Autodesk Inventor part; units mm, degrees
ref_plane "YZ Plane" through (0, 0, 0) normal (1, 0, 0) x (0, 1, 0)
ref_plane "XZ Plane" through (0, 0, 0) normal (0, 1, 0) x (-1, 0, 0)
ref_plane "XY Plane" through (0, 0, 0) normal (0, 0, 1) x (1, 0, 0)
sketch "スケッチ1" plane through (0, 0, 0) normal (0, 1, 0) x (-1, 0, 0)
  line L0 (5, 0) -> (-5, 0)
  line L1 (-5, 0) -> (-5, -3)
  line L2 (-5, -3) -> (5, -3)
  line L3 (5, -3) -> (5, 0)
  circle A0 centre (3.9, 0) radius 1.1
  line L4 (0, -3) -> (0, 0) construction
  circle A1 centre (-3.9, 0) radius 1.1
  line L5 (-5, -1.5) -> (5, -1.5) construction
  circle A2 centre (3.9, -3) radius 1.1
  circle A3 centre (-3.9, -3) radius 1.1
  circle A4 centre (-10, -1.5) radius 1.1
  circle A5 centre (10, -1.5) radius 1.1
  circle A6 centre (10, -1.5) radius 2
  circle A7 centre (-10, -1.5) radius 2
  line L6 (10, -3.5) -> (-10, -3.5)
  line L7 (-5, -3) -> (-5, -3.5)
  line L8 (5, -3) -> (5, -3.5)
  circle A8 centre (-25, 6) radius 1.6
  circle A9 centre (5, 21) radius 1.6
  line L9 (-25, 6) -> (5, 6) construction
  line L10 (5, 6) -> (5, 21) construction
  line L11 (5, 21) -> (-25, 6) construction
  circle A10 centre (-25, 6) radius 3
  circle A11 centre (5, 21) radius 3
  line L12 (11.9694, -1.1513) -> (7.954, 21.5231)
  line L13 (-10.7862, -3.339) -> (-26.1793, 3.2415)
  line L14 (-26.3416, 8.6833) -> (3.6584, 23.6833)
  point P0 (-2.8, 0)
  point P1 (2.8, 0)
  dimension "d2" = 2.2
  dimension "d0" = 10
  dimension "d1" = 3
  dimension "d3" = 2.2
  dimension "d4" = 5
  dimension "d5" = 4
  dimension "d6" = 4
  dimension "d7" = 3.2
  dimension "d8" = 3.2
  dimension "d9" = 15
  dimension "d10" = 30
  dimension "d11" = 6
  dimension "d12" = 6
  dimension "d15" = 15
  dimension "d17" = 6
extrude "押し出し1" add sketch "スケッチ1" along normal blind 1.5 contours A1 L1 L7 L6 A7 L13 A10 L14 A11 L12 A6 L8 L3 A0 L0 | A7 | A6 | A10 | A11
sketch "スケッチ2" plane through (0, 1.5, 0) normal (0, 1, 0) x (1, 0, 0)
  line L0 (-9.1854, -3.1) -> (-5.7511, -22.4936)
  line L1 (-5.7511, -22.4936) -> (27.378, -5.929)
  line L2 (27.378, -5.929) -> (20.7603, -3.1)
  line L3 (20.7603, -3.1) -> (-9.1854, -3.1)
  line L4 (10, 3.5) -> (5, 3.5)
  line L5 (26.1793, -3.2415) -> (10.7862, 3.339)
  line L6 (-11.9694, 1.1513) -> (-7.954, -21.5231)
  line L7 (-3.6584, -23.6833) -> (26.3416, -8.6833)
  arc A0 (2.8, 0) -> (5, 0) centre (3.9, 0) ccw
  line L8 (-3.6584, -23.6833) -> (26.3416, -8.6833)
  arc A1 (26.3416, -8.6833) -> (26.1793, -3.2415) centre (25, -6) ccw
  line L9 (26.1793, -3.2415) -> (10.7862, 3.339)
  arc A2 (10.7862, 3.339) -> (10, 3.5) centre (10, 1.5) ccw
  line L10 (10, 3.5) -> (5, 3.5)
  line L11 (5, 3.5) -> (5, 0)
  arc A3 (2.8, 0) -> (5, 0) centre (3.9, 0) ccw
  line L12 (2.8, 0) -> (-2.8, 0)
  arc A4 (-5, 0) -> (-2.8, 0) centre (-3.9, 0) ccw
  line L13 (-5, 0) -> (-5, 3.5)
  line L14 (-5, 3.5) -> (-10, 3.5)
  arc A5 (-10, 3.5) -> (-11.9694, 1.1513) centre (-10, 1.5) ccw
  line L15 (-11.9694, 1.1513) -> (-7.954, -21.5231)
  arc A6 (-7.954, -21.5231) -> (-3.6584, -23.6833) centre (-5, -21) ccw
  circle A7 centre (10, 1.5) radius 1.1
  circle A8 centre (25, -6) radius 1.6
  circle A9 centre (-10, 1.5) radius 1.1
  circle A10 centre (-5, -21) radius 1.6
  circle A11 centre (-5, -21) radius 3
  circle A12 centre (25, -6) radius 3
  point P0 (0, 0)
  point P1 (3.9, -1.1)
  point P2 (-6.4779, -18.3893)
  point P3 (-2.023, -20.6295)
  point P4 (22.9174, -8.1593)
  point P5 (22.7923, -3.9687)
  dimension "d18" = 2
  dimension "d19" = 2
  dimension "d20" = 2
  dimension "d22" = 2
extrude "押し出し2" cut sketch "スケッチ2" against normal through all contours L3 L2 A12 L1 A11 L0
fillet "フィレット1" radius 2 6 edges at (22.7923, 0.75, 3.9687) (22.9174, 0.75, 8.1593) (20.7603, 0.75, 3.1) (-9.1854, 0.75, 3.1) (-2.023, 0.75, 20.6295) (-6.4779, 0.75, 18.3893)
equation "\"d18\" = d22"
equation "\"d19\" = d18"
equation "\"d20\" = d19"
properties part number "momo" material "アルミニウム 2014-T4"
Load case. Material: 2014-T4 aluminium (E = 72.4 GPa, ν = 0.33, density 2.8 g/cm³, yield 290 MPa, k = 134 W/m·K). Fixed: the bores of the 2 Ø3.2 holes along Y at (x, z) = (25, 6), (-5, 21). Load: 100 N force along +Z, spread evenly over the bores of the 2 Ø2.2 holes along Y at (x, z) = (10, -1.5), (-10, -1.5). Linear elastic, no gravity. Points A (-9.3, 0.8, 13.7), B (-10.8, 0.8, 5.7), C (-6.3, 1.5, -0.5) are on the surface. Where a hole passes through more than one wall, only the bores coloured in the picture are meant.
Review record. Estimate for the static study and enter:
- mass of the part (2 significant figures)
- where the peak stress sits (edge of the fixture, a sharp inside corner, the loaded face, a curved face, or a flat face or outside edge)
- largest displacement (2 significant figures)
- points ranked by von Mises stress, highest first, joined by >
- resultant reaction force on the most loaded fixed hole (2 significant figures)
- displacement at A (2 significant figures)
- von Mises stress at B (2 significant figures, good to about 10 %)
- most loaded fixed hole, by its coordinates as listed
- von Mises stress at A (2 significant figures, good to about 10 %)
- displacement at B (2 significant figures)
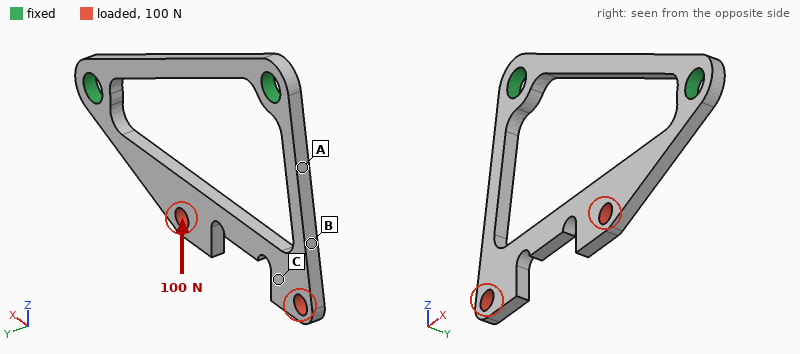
1.2 g
a curved face
73 µm
B > A > C
68 N
13 µm
64 MPa
(-5, 21)
25 MPa
22 µm
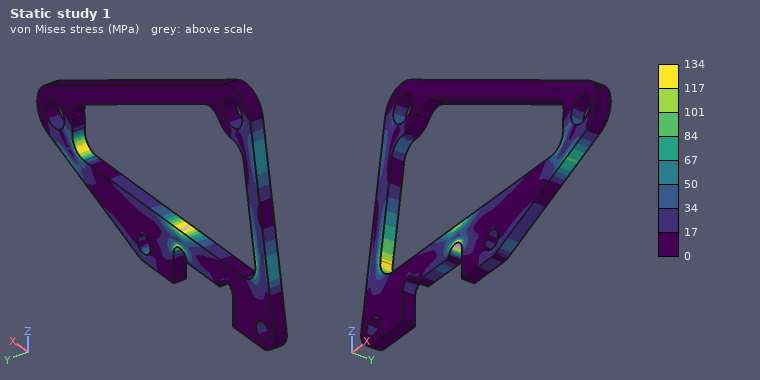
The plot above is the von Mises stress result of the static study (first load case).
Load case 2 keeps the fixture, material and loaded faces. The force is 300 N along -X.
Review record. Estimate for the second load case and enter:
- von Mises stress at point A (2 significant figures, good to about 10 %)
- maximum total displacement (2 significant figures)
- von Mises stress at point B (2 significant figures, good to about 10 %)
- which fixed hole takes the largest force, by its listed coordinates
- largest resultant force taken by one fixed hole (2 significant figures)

27 MPa
73 µm
61 MPa
(25, 6)
310 N
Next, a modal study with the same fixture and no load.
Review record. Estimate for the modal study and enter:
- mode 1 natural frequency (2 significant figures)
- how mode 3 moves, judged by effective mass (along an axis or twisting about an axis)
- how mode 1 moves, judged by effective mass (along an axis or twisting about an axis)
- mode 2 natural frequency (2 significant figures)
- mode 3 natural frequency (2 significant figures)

1700 Hz
along Z
along Y
4700 Hz
7500 Hz
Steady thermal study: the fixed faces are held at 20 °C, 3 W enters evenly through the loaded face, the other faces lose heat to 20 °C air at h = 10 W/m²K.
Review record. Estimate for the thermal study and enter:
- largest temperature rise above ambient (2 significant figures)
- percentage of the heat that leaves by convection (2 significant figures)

53 K
6.4 %
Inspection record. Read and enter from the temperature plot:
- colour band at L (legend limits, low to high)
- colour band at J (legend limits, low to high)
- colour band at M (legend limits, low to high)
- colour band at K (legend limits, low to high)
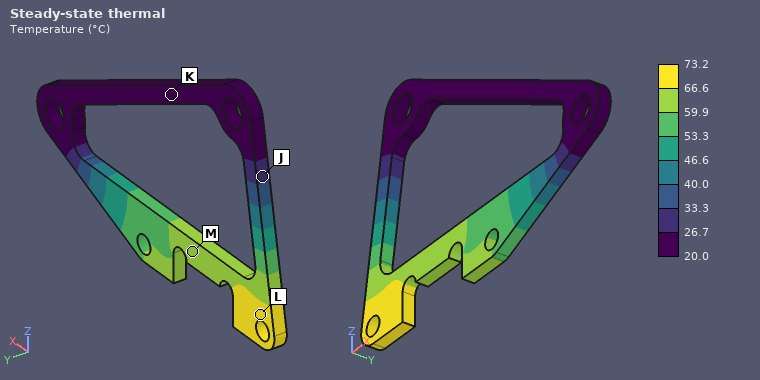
66.6 to 73.2 °C
26.7 to 33.3 °C
59.9 to 66.6 °C
20.0 to 26.7 °C
